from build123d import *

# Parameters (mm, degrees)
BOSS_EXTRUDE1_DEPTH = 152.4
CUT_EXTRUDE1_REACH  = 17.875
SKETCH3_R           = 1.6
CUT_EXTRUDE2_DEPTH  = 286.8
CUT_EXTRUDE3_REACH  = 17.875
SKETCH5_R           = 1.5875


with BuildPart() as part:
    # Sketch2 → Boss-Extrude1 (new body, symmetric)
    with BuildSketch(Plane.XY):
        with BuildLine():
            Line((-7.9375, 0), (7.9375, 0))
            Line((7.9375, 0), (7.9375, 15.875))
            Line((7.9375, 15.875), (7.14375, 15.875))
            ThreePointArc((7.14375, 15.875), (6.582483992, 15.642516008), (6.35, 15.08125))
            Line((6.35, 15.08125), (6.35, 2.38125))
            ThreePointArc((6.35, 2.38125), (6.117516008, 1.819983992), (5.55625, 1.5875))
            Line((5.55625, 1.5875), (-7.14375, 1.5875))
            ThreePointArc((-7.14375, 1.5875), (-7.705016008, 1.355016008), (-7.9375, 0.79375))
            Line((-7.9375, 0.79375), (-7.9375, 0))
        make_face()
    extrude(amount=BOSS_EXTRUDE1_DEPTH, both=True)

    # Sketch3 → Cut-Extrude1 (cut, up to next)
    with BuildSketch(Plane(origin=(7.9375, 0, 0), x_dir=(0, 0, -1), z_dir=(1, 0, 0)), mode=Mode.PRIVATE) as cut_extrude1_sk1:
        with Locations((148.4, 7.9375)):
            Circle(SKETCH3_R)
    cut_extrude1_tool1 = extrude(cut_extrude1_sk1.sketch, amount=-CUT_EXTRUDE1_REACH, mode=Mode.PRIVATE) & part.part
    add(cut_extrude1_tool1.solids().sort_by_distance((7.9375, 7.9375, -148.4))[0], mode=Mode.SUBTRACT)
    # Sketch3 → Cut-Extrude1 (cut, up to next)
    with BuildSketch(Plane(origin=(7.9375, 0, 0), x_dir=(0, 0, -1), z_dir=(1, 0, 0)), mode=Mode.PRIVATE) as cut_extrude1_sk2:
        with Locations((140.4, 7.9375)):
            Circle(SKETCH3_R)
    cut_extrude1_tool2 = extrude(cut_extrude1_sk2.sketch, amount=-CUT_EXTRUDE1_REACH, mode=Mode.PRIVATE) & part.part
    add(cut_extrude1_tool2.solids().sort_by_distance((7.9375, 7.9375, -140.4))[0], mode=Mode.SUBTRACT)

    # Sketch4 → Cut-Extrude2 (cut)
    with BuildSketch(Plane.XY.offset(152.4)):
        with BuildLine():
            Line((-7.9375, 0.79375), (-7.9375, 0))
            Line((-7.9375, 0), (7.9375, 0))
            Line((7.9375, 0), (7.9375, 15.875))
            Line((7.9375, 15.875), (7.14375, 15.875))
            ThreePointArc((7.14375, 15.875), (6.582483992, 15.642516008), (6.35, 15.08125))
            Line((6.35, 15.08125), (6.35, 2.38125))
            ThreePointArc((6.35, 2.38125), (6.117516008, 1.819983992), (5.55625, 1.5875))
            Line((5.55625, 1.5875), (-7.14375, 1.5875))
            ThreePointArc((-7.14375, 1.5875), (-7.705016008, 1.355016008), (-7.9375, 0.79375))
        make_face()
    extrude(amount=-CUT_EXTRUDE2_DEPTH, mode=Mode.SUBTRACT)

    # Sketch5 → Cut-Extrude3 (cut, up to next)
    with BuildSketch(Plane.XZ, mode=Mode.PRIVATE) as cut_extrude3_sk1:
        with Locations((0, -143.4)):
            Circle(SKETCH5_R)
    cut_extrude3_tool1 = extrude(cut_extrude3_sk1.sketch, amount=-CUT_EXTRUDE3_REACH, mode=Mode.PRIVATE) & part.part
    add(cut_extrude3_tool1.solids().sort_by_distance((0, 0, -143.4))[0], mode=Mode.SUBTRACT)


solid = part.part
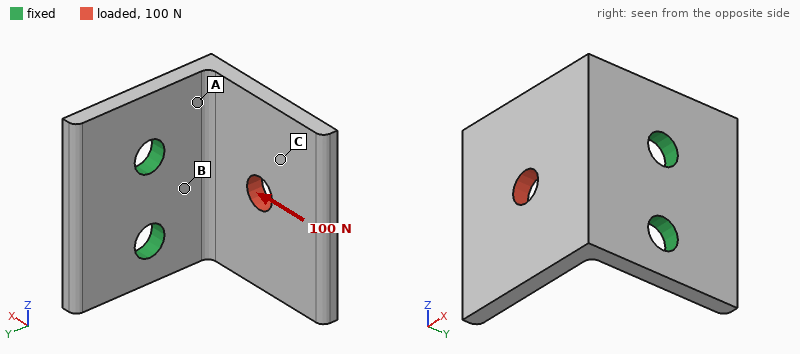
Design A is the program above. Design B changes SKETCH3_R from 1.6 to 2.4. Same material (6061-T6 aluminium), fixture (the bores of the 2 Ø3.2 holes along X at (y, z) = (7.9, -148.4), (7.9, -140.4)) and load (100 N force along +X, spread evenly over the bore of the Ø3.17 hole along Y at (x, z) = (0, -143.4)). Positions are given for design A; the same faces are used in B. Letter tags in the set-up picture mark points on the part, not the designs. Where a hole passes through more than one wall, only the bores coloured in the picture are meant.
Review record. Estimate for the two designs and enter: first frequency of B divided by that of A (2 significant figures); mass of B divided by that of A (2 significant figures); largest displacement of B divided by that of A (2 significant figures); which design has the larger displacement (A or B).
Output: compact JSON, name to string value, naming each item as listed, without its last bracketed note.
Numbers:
{"first frequency of B divided by that of A": "1.1", "mass of B divided by that of A": "0.96", "largest displacement of B divided by that of A": "0.72", "which design has the larger displacement": "A"}
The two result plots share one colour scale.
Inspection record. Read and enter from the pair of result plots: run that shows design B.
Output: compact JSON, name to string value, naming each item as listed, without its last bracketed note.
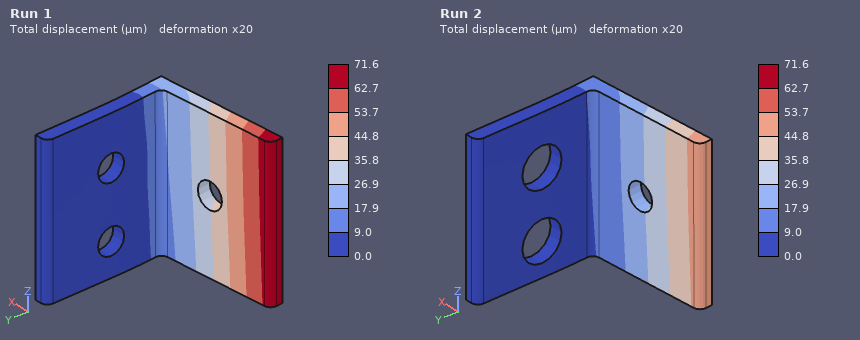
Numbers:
{"run that shows design B": "Run 2"}
